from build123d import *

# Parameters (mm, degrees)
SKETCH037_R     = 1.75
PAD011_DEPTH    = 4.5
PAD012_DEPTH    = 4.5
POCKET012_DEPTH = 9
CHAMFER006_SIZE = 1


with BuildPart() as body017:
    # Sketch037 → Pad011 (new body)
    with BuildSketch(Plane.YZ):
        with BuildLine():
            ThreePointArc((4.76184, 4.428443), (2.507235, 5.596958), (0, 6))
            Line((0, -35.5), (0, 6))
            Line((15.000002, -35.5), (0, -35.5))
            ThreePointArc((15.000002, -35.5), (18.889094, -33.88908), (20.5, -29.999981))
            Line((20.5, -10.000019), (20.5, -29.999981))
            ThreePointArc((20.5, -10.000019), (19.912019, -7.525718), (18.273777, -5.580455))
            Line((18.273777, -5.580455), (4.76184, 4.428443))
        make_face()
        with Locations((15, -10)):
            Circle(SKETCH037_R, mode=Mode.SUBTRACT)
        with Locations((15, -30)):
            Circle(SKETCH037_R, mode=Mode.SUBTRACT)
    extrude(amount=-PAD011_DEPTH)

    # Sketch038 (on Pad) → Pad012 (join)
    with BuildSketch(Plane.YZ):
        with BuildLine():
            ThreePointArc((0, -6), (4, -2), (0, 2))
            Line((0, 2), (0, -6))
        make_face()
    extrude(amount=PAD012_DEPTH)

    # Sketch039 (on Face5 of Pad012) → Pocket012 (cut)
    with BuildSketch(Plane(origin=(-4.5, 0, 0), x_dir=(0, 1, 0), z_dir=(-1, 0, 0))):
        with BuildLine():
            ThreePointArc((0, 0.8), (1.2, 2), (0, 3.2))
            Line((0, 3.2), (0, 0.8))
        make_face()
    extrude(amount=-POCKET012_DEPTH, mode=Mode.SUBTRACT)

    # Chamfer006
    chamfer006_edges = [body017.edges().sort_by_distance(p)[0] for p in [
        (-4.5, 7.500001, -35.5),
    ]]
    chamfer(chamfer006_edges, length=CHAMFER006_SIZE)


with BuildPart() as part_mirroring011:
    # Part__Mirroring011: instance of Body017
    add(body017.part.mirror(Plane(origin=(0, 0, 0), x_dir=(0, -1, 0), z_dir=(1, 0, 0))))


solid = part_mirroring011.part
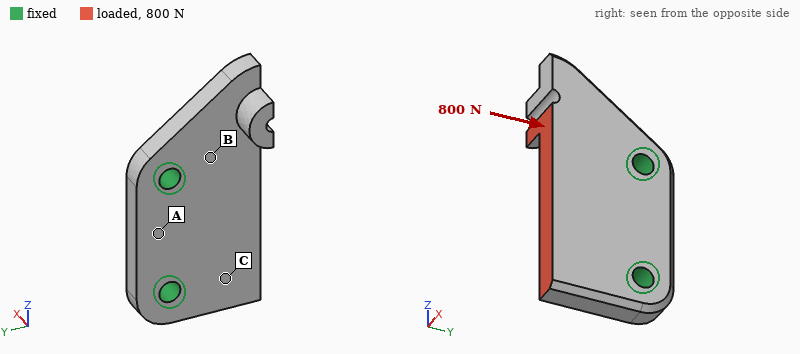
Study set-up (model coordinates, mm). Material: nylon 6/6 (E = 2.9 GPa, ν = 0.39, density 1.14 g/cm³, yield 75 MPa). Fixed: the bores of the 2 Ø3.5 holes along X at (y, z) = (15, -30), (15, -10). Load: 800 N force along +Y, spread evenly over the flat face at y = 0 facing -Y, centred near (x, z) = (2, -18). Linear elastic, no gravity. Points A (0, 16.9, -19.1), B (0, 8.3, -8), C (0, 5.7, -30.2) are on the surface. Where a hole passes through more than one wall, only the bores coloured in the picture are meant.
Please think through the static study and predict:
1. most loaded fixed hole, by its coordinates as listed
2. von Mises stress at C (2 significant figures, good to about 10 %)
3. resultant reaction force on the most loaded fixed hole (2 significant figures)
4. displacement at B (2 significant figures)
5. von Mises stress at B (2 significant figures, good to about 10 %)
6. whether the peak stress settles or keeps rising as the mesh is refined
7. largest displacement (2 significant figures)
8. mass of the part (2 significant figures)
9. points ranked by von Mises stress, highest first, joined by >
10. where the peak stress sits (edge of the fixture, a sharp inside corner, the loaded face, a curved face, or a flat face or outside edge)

(15, -10)
6.1 MPa
470 N
0.038 mm
13 MPa
keeps rising
0.22 mm
3.7 g
B > C > A
edge of the fixture
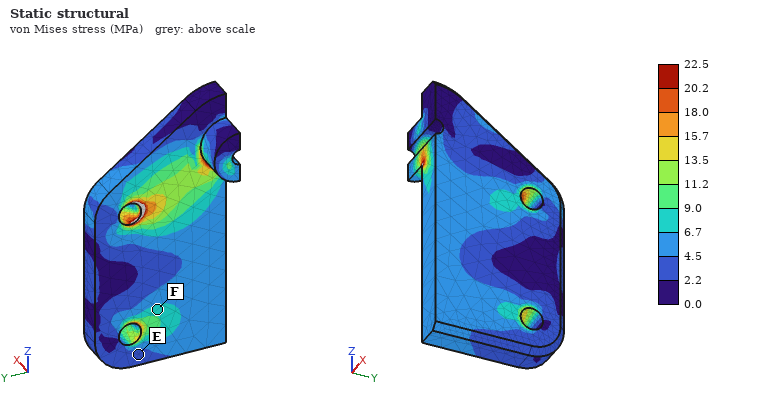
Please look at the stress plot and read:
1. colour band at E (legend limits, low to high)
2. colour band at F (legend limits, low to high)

2.2 to 4.5 MPa
6.7 to 9.0 MPa
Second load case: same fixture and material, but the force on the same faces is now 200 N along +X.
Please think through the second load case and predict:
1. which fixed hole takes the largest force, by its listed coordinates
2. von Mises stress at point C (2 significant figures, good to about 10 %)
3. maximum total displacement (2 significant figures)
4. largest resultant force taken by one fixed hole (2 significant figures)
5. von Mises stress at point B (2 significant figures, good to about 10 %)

(15, -10)
9.9 MPa
0.41 mm
120 N
14 MPa
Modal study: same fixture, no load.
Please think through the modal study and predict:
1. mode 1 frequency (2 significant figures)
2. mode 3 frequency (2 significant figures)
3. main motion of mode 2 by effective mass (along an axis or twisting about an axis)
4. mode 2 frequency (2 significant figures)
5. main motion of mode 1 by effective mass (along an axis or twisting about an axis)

3400 Hz
7800 Hz
along X
4900 Hz
along X
